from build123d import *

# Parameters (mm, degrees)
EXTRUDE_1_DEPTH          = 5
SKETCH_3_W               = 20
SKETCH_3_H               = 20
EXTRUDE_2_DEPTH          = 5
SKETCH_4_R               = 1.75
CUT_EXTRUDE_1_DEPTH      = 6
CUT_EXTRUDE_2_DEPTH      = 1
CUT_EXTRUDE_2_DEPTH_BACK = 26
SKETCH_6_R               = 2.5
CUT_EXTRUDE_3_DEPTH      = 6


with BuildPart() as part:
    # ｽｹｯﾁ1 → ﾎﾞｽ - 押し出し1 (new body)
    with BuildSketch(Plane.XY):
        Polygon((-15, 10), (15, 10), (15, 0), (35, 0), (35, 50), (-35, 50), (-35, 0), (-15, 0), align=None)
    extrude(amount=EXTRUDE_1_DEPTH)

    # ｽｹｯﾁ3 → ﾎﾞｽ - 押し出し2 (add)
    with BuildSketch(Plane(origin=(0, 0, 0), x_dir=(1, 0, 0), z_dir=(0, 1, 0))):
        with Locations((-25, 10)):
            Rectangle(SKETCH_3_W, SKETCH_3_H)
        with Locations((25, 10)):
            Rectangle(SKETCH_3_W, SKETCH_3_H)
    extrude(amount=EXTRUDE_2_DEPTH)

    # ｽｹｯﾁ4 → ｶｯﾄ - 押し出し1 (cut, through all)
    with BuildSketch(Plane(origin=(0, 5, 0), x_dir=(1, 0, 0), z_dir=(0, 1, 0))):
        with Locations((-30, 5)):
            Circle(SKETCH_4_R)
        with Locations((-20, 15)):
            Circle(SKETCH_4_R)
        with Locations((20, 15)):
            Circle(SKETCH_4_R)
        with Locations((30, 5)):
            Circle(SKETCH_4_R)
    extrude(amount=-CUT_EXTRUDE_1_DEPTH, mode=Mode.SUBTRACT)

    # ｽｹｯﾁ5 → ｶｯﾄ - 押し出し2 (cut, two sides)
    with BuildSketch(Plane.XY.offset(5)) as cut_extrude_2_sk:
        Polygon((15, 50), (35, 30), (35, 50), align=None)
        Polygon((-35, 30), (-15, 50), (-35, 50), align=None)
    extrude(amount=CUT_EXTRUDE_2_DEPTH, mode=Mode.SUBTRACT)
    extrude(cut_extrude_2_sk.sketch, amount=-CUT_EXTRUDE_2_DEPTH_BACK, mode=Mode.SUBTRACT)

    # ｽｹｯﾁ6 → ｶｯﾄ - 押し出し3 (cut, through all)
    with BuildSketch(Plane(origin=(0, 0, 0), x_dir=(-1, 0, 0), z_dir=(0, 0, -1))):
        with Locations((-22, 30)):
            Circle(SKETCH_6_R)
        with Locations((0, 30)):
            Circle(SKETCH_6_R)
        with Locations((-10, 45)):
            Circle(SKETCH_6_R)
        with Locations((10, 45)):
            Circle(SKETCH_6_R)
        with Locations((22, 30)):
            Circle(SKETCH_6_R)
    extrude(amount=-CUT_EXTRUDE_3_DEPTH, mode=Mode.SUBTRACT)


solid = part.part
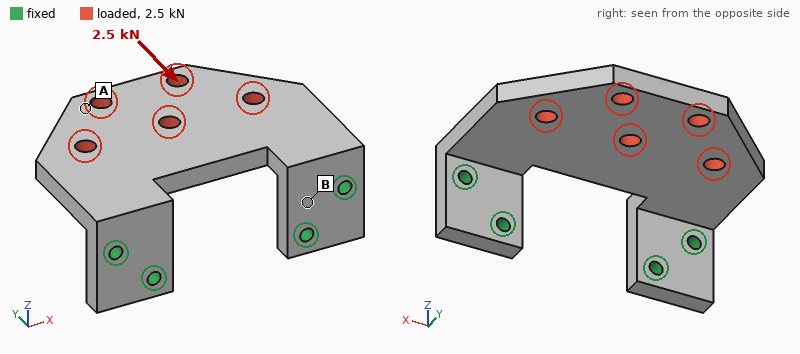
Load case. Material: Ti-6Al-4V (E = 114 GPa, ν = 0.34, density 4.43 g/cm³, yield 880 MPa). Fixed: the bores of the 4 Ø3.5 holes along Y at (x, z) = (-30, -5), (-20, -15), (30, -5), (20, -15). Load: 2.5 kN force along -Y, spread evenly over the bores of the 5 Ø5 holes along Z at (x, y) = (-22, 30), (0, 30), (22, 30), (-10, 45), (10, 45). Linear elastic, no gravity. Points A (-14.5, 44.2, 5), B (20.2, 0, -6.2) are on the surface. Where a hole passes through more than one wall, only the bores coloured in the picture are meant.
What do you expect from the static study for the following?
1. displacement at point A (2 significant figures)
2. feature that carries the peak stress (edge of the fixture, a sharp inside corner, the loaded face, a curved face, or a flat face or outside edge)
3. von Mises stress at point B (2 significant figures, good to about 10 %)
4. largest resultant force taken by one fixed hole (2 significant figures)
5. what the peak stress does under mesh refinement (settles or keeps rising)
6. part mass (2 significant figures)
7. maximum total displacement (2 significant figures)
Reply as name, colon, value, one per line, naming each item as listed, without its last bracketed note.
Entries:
displacement at point A: 79 µm
feature that carries the peak stress: edge of the fixture
von Mises stress at point B: 31 MPa
largest resultant force taken by one fixed hole: 1.5 kN
what the peak stress does under mesh refinement: keeps rising
part mass: 77 g
maximum total displacement: 90 µm
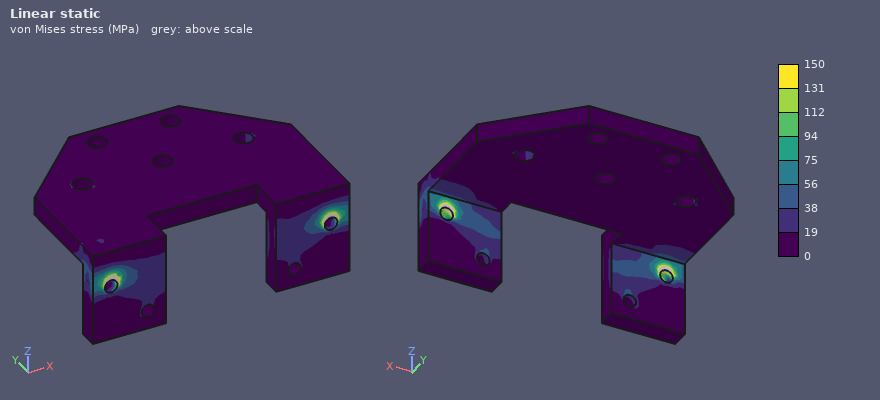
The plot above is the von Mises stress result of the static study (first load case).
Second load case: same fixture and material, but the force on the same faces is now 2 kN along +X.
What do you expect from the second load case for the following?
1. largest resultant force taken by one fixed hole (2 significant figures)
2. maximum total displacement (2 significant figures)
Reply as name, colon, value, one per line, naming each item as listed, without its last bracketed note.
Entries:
largest resultant force taken by one fixed hole: 1.6 kN
maximum total displacement: 32 µm
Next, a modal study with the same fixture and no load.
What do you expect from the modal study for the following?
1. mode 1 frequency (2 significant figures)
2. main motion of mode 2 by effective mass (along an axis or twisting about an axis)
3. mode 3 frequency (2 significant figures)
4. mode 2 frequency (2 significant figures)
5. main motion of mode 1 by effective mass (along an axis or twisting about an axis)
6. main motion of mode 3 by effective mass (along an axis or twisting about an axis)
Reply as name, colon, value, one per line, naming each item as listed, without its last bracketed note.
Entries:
mode 1 frequency: 1400 Hz
main motion of mode 2 by effective mass: twisting about Y
mode 3 frequency: 7400 Hz
mode 2 frequency: 4000 Hz
main motion of mode 1 by effective mass: along Z
main motion of mode 3 by effective mass: along Y
